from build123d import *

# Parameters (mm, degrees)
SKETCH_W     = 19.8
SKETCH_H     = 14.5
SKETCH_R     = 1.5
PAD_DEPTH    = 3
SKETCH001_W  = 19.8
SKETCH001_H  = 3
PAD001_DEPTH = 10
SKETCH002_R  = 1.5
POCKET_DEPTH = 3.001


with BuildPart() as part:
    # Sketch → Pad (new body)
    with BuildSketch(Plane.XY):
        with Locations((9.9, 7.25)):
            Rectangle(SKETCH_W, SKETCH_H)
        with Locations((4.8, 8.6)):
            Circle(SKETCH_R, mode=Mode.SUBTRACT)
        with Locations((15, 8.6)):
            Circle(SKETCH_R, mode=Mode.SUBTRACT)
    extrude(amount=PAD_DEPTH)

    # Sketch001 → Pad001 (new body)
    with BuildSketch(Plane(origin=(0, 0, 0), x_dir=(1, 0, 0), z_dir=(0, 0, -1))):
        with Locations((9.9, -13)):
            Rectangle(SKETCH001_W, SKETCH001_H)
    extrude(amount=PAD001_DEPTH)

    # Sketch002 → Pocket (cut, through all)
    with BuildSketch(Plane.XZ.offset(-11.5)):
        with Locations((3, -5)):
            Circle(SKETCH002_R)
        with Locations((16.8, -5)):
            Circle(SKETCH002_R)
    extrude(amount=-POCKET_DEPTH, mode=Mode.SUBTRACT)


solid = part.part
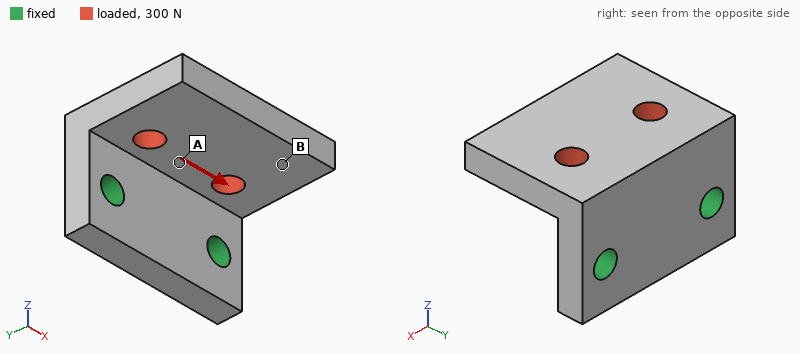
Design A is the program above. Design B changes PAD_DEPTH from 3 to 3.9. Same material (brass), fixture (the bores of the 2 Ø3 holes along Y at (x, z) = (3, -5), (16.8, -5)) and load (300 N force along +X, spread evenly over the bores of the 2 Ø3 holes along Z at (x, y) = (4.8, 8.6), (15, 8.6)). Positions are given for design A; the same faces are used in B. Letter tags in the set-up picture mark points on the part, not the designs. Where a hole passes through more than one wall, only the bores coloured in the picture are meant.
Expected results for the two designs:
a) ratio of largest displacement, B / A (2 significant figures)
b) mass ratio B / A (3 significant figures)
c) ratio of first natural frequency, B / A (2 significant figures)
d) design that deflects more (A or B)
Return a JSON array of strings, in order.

["0.91", "1.18", "0.92", "A"]
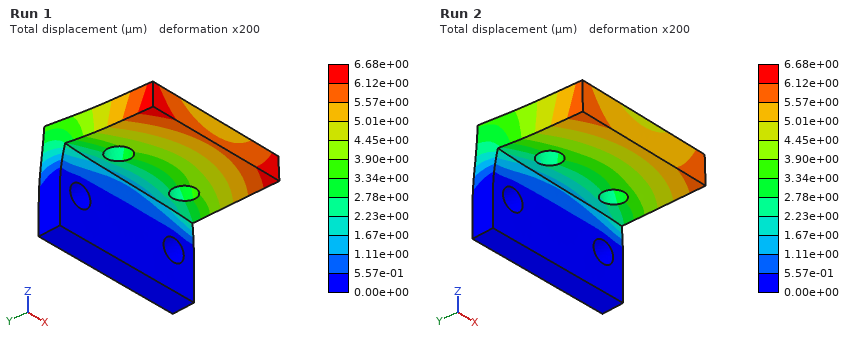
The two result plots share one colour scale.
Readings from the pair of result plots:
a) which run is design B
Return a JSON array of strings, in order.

["Run 2"]
